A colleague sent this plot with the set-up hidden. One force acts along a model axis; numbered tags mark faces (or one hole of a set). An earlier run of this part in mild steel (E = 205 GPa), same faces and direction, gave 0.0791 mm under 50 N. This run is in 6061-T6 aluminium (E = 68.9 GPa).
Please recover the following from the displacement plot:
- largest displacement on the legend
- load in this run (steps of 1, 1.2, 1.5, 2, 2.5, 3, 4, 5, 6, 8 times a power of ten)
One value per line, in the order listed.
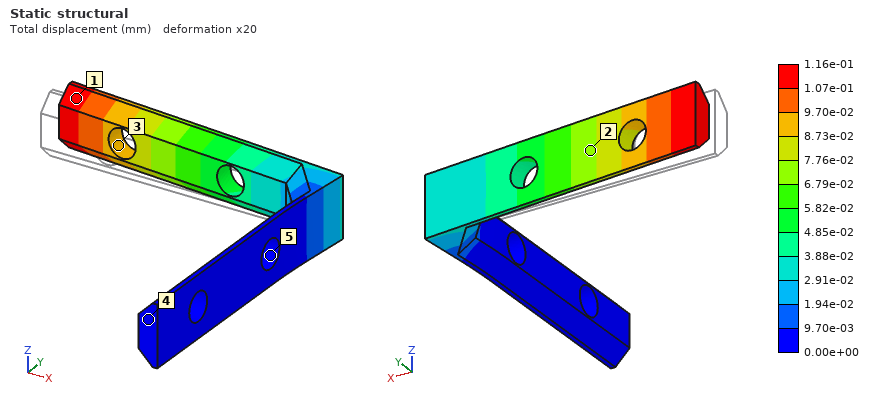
1.16e-01 mm
25 N
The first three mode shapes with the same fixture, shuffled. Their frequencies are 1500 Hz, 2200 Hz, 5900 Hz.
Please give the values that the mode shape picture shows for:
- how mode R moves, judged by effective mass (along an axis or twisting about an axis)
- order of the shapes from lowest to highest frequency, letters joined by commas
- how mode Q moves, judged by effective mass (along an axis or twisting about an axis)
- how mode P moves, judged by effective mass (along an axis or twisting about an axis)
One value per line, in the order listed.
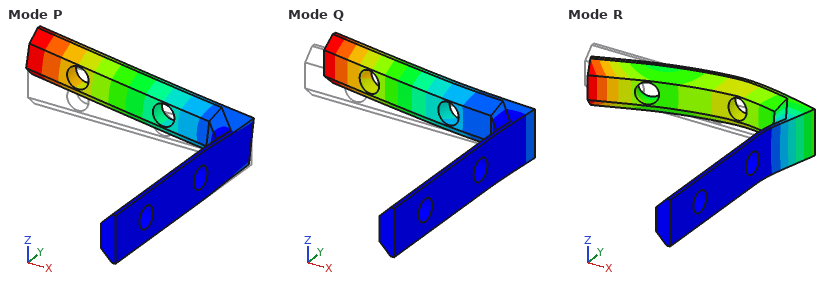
along X
Q, P, R
along Y
along Z
